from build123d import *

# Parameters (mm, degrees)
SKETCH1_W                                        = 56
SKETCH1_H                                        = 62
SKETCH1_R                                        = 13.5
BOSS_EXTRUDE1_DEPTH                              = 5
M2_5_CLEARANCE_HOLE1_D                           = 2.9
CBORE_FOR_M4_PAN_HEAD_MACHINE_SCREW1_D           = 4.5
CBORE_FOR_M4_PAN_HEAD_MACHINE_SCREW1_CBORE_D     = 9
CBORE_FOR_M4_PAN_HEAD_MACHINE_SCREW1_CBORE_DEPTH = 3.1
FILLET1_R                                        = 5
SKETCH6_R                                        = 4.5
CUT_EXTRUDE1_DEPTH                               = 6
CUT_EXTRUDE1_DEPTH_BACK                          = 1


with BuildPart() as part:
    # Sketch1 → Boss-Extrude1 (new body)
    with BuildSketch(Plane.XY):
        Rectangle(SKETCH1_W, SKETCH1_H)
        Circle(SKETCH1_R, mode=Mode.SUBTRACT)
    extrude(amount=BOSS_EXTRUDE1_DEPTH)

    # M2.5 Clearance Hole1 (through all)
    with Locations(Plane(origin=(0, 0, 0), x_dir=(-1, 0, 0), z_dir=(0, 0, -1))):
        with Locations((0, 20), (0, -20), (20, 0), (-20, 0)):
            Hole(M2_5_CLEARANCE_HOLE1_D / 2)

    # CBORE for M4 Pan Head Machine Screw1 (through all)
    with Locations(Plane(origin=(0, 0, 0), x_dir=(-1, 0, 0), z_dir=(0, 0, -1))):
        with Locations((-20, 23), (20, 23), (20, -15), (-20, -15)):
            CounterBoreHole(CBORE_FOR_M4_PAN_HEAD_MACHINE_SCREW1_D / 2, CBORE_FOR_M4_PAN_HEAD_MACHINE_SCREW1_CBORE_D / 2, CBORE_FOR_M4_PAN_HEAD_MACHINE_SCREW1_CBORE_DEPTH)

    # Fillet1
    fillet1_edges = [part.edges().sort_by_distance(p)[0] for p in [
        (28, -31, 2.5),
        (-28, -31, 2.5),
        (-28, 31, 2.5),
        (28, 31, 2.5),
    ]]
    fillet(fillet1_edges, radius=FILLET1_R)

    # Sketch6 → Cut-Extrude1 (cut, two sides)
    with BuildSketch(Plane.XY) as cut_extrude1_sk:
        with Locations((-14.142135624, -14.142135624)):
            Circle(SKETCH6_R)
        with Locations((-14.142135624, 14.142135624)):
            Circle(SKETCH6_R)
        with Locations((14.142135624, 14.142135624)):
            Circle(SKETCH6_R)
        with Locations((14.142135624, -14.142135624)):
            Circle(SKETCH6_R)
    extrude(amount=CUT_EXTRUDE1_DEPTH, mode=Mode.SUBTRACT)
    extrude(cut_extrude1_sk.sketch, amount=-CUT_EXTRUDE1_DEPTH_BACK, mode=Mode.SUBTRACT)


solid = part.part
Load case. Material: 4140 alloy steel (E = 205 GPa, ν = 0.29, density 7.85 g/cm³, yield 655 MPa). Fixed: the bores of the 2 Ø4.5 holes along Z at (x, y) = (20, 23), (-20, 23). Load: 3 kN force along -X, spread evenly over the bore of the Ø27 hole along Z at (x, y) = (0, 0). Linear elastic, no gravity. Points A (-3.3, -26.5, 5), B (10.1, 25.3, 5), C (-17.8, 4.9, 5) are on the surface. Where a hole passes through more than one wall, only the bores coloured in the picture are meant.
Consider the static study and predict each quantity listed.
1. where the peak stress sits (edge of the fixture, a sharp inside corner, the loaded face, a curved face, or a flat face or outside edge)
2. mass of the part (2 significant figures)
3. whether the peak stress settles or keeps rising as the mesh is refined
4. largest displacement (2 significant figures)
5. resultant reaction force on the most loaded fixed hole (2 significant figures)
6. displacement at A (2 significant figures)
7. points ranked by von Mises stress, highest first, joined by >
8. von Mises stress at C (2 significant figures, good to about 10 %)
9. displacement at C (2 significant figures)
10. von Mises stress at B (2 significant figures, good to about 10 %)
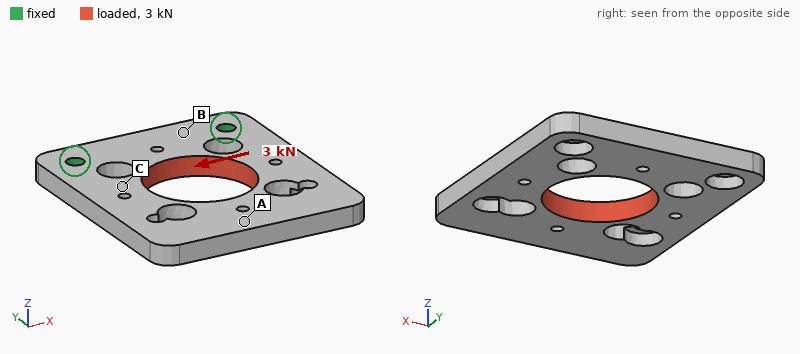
edge of the fixture
96 g
keeps rising
31 µm
2.2 kN
27 µm
C > B > A
45 MPa
13 µm
28 MPa
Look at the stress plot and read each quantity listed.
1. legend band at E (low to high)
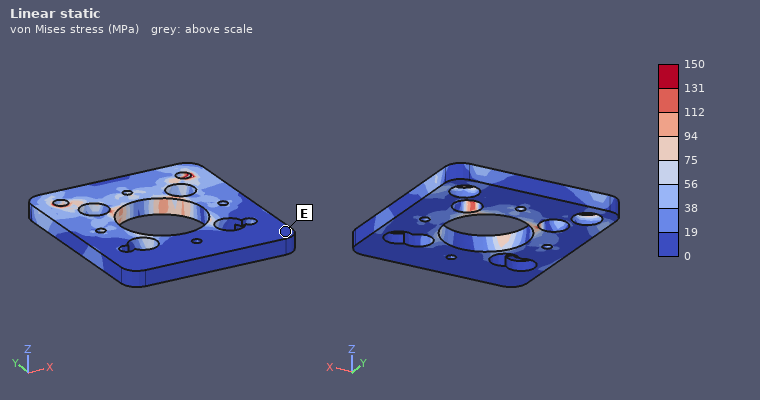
0 to 19 MPa
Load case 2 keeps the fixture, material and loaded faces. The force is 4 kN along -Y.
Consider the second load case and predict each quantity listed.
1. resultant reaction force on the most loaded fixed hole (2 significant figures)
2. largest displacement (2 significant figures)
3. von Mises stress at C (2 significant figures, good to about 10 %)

2.0 kN
77 µm
30 MPa
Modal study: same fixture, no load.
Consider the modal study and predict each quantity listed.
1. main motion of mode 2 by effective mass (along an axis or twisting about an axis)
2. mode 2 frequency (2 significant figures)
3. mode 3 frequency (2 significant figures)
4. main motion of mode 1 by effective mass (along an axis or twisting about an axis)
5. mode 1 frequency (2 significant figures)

twisting about Y
2300 Hz
5600 Hz
along Z
830 Hz
